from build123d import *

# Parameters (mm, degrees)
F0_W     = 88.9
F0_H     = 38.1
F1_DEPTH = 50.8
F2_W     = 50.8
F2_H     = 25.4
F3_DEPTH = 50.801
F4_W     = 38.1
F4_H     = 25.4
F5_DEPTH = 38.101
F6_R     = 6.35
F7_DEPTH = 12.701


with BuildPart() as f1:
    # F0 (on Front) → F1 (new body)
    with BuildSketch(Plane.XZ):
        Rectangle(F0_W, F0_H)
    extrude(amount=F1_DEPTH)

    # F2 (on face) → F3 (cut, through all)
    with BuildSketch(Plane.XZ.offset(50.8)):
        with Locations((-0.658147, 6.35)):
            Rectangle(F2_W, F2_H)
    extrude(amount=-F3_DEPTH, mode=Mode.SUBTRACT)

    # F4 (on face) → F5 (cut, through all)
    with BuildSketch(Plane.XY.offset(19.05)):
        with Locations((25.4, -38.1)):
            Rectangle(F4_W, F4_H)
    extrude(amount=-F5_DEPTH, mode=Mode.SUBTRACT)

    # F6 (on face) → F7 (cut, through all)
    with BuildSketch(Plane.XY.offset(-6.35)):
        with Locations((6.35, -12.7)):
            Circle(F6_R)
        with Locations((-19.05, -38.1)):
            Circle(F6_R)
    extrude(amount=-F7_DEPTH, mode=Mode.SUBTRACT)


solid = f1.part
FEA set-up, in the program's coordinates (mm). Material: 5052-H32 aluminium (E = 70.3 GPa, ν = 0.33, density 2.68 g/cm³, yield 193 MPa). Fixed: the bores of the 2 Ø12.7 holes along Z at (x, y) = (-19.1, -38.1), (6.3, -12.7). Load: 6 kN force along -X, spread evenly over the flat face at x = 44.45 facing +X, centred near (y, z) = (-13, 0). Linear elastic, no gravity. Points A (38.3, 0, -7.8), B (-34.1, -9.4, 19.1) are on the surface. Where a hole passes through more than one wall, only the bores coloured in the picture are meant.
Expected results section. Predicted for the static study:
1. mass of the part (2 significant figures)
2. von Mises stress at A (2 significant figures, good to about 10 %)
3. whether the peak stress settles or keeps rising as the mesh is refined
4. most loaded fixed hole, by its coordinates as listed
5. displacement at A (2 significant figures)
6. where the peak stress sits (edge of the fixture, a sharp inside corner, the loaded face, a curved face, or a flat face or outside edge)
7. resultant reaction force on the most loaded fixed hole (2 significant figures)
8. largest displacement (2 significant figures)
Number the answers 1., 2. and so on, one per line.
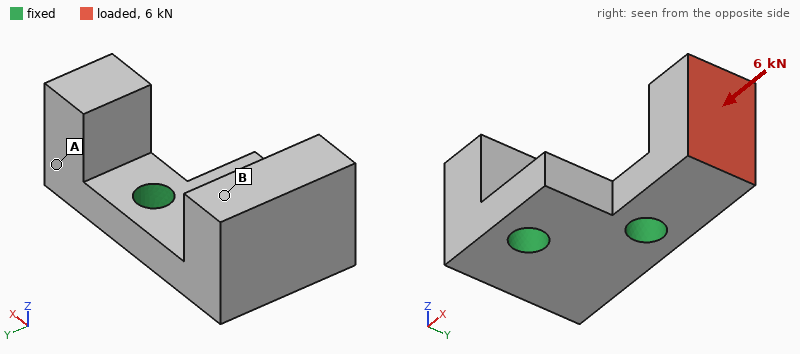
1. 210 g
2. 24 MPa
3. keeps rising
4. (6.3, -12.7)
5. 0.095 mm
6. edge of the fixture
7. 5.8 kN
8. 0.21 mm
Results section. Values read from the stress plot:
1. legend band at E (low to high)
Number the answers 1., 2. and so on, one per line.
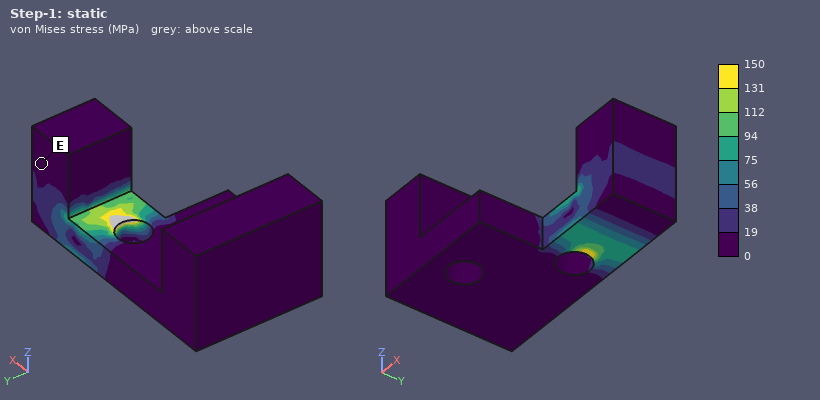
1. 0 to 19 MPa
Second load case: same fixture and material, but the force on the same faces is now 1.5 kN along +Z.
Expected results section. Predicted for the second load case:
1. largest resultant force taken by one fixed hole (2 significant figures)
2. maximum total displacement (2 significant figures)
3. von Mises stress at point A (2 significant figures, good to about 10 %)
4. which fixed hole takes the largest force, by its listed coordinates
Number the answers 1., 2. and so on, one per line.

1. 1.6 kN
2. 0.10 mm
3. 10 MPa
4. (6.3, -12.7)
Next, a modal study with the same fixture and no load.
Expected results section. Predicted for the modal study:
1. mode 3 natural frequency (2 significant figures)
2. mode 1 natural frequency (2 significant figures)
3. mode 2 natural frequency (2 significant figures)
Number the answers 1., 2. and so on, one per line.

1. 4800 Hz
2. 3600 Hz
3. 4700 Hz
